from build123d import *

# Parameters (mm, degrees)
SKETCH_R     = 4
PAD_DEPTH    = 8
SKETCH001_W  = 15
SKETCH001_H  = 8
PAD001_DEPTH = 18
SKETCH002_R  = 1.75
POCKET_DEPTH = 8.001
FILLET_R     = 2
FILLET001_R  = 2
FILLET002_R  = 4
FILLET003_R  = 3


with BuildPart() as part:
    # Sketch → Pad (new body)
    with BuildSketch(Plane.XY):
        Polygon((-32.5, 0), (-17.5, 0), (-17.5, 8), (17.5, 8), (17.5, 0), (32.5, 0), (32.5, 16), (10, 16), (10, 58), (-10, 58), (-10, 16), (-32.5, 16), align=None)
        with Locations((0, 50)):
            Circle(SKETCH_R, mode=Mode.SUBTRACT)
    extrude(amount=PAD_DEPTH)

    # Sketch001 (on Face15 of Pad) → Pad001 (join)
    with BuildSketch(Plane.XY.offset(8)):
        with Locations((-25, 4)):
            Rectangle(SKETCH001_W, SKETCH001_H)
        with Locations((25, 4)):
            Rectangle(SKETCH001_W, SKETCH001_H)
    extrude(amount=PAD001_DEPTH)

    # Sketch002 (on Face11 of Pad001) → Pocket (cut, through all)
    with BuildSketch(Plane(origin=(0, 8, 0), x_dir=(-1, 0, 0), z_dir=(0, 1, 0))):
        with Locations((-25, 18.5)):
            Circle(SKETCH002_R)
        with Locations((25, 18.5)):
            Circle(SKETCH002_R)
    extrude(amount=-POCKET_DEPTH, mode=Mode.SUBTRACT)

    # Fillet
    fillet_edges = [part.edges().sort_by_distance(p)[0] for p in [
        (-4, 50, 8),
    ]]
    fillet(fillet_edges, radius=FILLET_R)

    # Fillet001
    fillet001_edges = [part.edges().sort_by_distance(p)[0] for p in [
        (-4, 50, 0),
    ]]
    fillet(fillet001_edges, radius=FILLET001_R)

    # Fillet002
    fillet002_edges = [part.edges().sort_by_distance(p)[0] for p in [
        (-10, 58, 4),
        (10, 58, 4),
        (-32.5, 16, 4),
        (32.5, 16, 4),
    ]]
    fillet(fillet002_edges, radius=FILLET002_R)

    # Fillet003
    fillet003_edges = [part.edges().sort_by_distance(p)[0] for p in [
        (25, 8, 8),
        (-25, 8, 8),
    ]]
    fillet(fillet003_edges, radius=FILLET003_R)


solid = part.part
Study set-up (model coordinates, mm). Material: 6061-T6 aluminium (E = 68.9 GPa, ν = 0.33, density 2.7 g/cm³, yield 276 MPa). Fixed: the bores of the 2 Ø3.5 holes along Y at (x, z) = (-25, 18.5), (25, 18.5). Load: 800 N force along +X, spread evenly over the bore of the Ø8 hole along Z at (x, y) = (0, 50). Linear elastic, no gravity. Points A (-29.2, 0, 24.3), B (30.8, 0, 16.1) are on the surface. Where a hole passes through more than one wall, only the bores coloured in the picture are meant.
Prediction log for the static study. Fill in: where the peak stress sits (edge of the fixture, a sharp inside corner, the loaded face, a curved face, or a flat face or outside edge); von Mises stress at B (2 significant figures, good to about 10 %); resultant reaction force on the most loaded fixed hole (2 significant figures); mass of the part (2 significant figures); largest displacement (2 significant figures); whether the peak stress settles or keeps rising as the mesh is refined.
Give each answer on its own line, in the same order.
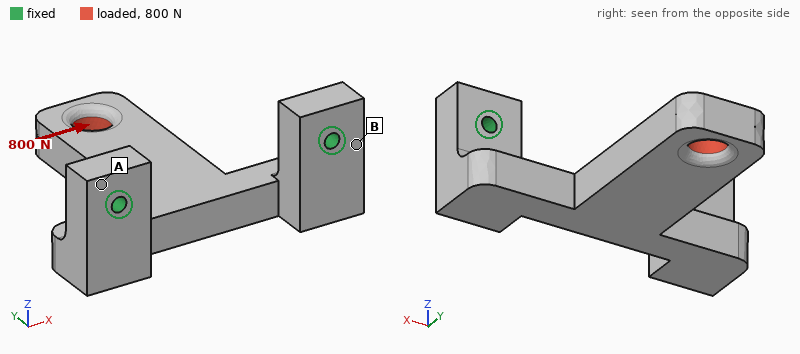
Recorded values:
edge of the fixture
30 MPa
900 N
44 g
0.17 mm
keeps rising
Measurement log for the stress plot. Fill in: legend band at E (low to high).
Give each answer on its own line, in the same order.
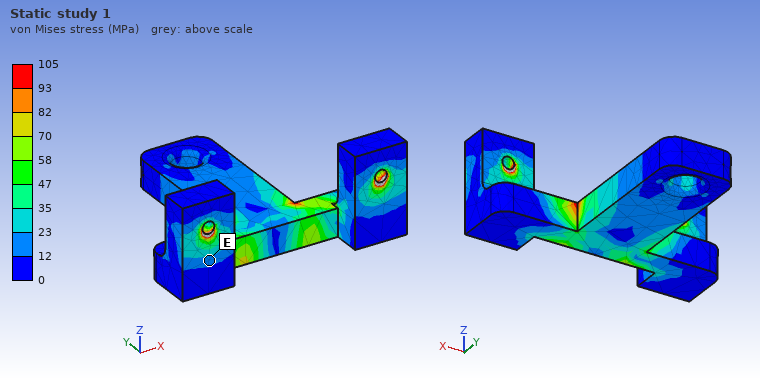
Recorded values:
12 to 23 MPa
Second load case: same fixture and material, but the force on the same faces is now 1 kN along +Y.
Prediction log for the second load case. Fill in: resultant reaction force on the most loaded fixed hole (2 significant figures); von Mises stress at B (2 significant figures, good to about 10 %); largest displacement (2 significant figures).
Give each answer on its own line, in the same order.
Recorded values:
550 N
27 MPa
94 µm
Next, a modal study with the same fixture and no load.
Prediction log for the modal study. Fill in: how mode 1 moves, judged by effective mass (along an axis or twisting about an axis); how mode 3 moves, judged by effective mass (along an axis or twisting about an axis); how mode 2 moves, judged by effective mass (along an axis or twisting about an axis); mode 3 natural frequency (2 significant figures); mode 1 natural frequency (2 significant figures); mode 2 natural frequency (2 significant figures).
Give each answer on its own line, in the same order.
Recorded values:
along Z
along Y
along X
5600 Hz
1500 Hz
4100 Hz
